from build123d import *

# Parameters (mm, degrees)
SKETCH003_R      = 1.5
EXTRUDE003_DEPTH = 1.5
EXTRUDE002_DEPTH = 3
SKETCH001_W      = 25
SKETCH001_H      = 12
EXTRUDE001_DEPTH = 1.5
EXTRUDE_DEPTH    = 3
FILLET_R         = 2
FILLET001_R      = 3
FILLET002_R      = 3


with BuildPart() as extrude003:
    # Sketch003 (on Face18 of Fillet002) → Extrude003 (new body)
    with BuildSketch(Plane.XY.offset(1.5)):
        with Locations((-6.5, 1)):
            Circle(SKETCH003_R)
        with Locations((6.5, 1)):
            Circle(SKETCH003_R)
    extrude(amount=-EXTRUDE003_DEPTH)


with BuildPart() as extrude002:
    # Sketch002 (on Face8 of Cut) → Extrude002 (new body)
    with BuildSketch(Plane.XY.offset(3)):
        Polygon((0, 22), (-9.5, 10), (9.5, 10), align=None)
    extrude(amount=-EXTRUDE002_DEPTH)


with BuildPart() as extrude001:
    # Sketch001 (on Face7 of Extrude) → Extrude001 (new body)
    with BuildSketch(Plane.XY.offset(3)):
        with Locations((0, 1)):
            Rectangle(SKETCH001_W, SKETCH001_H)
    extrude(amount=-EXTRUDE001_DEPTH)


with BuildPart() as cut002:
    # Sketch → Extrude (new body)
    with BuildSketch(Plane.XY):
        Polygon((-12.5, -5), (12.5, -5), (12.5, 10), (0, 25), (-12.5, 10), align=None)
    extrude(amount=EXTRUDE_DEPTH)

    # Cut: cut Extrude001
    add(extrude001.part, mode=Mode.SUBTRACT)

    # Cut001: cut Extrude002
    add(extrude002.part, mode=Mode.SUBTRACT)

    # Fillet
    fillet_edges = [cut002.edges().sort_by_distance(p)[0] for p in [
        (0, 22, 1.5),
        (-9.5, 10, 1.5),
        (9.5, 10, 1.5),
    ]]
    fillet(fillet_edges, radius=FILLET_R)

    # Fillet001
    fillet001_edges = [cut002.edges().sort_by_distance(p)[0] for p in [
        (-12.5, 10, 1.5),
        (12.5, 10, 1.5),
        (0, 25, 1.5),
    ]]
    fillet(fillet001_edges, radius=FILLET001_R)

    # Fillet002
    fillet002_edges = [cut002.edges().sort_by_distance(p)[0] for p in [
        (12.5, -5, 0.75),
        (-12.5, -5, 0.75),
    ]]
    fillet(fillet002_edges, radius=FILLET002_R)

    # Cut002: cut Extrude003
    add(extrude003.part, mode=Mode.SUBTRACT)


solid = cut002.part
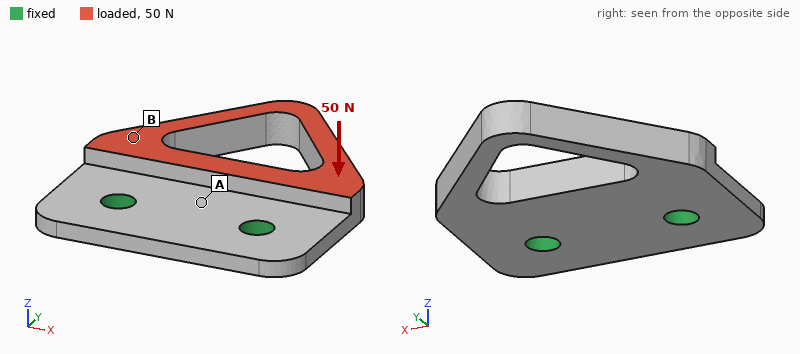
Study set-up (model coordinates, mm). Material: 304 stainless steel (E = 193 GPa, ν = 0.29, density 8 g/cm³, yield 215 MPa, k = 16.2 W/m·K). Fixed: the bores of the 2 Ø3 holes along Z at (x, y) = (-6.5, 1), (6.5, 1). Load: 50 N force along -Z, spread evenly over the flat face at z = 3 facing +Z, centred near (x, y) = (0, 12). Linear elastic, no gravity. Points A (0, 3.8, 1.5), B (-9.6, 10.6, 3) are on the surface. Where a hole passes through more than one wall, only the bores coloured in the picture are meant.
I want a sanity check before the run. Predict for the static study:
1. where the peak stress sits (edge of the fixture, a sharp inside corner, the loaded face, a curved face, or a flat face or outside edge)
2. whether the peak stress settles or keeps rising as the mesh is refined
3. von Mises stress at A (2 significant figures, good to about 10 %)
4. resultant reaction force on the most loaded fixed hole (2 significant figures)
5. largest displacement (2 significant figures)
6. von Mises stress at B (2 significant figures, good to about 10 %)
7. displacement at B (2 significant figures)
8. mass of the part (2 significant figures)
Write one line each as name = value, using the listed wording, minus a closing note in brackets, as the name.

where the peak stress sits = edge of the fixture
whether the peak stress settles or keeps rising as the mesh is refined = keeps rising
von Mises stress at A = 31 MPa
resultant reaction force on the most loaded fixed hole = 25 N
largest displacement = 38 µm
von Mises stress at B = 11 MPa
displacement at B = 12 µm
mass of the part = 7.1 g
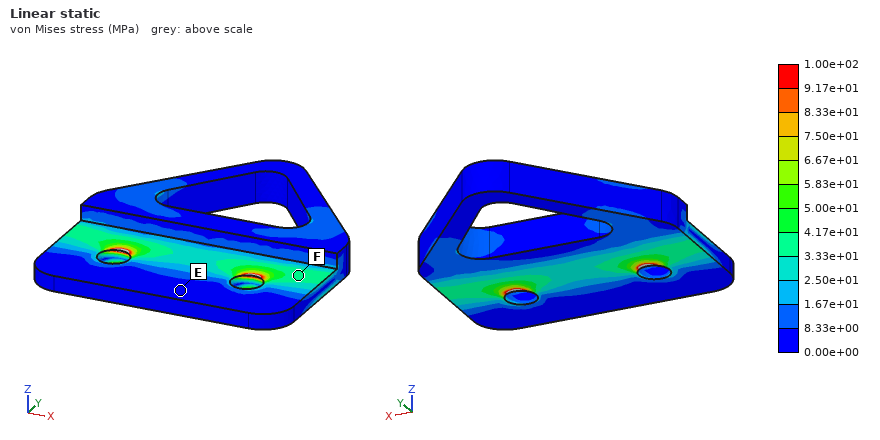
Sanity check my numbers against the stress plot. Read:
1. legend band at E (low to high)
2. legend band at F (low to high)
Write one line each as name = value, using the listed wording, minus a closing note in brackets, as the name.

legend band at E = 0.00e+00 to 8.33e+00 MPa
legend band at F = 3.33e+01 to 4.17e+01 MPa
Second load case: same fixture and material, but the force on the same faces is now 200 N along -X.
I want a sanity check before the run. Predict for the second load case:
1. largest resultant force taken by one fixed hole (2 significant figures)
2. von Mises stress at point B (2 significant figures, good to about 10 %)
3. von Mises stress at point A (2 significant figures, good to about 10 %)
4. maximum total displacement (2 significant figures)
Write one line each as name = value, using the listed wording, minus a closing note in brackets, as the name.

largest resultant force taken by one fixed hole = 170 N
von Mises stress at point B = 13 MPa
von Mises stress at point A = 21 MPa
maximum total displacement = 5.9 µm
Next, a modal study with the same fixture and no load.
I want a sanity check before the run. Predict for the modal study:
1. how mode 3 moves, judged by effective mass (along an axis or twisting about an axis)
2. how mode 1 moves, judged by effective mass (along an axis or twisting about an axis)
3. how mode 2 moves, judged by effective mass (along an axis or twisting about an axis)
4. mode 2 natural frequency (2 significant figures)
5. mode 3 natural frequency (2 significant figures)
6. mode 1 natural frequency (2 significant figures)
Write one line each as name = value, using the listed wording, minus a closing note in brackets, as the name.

how mode 3 moves, judged by effective mass = along Z
how mode 1 moves, judged by effective mass = along Z
how mode 2 moves, judged by effective mass = twisting about Y
mode 2 natural frequency = 11 kHz
mode 3 natural frequency = 17 kHz
mode 1 natural frequency = 4000 Hz
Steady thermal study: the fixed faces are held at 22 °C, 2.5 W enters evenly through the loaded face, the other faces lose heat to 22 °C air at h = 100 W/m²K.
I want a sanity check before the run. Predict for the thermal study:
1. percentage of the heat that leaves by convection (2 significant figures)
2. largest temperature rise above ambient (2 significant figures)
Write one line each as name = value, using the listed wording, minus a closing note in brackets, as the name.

percentage of the heat that leaves by convection = 51 %
largest temperature rise above ambient = 32 K
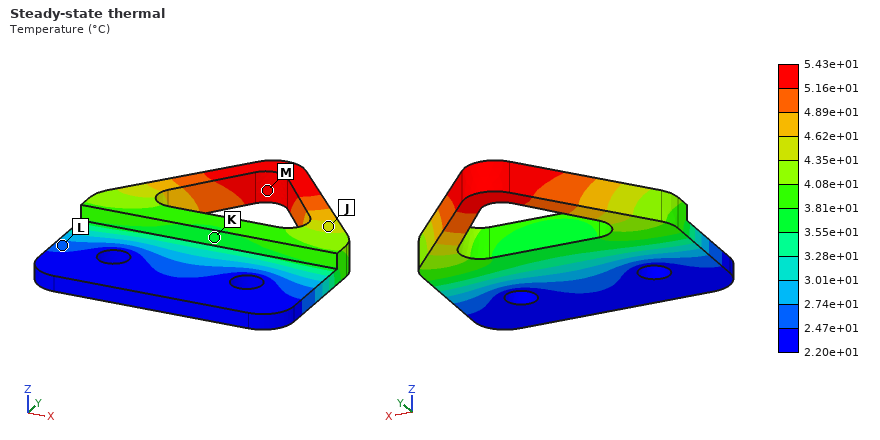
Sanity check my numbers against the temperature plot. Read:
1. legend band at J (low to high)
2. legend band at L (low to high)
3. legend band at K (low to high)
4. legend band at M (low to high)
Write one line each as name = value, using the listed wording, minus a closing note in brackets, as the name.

legend band at J = 4.35e+01 to 4.62e+01 °C
legend band at L = 2.47e+01 to 2.74e+01 °C
legend band at K = 3.55e+01 to 3.81e+01 °C
legend band at M = 5.16e+01 to 5.43e+01 °C
